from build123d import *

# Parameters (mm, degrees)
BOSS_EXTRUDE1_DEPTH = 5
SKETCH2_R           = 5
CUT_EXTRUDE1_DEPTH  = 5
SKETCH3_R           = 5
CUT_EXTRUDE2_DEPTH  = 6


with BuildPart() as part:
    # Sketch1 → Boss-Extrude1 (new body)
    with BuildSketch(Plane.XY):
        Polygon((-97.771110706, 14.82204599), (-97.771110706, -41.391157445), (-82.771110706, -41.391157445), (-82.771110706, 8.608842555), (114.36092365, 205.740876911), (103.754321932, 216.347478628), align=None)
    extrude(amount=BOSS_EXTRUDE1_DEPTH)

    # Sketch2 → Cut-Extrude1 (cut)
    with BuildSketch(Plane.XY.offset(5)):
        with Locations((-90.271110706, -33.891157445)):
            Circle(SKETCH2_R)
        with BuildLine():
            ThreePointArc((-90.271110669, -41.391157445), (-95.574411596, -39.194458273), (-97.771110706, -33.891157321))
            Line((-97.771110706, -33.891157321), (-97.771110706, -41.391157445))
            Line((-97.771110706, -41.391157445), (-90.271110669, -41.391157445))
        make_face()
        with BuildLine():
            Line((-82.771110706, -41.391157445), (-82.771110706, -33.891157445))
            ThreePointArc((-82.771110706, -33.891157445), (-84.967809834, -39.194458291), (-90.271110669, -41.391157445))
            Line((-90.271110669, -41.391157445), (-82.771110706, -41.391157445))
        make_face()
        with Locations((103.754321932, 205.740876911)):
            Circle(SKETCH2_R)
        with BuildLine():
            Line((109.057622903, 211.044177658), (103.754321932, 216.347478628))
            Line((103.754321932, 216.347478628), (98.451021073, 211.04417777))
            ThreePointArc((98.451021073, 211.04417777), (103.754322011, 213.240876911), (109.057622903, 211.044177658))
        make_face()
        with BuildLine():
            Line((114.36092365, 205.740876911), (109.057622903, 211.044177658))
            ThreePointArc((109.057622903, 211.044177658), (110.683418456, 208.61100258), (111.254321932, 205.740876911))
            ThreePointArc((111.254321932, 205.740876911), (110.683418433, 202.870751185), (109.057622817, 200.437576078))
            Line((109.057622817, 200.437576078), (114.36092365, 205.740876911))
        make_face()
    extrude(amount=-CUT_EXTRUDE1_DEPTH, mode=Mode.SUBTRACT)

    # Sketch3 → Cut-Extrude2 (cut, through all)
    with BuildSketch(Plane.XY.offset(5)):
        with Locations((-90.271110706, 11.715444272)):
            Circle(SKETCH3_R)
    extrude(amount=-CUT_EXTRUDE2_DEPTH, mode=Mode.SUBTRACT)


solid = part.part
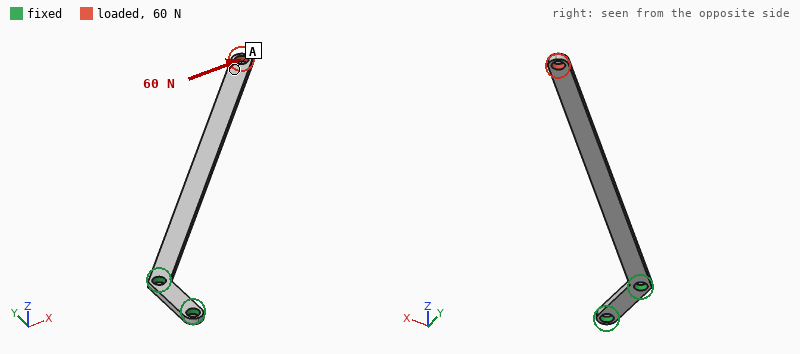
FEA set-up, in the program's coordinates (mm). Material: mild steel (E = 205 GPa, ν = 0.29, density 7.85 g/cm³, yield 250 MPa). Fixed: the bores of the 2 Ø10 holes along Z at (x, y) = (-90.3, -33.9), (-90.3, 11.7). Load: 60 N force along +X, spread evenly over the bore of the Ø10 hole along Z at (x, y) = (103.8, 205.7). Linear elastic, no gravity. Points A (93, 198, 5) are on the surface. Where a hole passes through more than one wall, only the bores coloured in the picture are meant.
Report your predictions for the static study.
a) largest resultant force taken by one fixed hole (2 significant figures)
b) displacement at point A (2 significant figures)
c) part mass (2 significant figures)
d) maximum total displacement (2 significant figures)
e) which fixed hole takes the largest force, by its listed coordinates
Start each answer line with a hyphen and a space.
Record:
- 85 N
- 0.93 mm
- 190 g
- 1.0 mm
- (-90.3, 11.7)
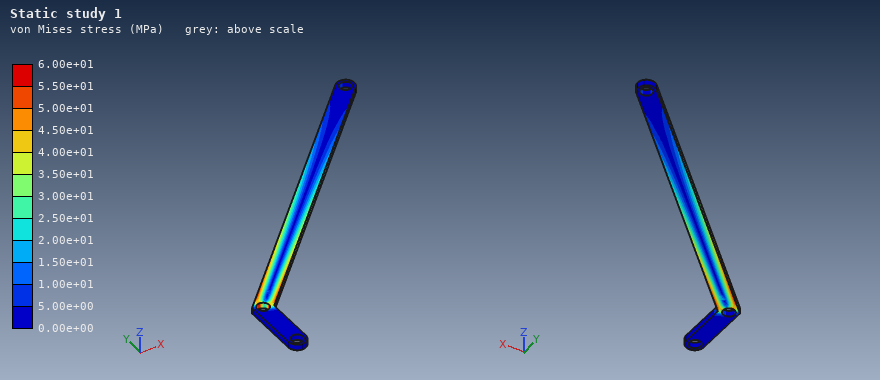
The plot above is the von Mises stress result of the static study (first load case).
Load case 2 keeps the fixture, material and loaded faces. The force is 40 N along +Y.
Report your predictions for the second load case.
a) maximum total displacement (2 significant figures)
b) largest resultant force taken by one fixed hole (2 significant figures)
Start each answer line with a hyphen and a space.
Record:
- 0.69 mm
- 25 N
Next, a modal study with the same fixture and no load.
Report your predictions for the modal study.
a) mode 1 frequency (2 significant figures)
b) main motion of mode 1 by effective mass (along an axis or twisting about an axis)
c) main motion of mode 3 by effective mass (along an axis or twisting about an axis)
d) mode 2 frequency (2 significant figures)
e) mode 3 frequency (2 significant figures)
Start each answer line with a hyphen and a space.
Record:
- 56 Hz
- along Z
- along Z
- 170 Hz
- 350 Hz
